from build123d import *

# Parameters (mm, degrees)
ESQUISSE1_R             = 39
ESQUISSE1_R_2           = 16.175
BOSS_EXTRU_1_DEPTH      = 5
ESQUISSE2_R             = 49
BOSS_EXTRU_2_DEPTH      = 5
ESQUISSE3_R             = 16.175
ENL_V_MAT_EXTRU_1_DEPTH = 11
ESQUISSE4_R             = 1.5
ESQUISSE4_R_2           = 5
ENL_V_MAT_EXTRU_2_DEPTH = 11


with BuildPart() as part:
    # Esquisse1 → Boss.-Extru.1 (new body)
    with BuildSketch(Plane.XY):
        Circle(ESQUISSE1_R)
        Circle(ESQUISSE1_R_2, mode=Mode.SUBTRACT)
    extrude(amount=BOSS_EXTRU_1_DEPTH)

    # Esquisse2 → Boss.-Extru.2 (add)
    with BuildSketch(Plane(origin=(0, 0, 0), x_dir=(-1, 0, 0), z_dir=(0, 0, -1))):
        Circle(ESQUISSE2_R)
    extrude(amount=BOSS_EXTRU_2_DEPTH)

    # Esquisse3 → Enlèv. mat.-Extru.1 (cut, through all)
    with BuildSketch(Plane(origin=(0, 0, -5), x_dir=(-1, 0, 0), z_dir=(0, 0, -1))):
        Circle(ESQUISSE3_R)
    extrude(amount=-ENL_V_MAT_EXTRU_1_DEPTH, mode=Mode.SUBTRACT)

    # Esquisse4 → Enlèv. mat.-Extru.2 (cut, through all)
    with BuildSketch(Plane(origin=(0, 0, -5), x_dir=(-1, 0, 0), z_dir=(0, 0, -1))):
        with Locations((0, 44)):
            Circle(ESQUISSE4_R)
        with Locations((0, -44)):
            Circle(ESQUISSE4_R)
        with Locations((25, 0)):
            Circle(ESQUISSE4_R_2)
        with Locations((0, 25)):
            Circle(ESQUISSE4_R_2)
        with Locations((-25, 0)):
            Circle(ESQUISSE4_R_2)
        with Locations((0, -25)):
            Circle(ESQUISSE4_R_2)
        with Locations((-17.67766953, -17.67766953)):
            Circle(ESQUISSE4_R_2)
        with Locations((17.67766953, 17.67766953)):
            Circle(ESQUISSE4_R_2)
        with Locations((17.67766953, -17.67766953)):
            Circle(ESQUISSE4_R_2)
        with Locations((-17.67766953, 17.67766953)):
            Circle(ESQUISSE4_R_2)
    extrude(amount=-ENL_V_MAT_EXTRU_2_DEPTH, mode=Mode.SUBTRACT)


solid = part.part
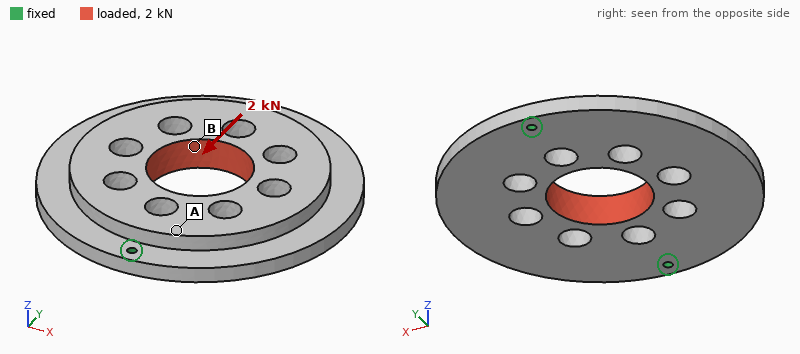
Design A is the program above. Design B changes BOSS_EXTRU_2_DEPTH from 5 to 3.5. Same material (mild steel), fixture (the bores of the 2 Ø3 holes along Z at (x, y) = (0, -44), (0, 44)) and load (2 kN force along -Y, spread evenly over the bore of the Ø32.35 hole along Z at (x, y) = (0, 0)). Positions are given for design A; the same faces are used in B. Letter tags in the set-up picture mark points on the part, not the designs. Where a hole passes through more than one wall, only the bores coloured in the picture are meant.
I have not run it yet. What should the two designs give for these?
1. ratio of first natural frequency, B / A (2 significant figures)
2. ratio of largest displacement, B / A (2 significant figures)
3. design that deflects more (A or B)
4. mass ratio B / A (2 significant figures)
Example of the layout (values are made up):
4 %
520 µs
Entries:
0.77
1.3
B
0.81
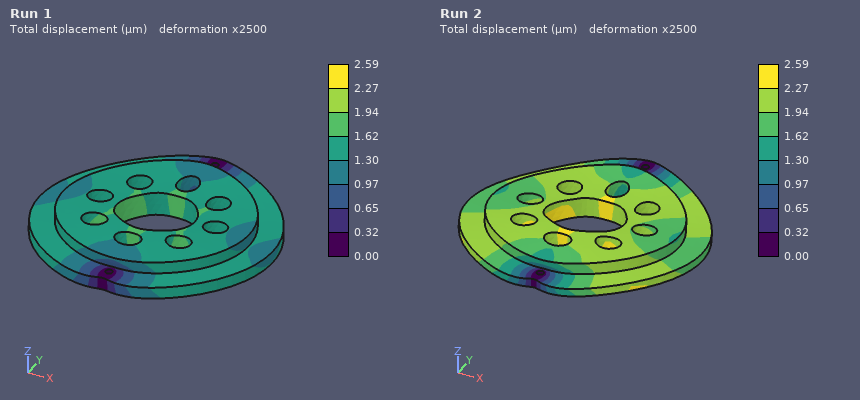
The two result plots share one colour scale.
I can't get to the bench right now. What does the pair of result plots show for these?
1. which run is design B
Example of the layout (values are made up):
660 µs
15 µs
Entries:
Run 2
